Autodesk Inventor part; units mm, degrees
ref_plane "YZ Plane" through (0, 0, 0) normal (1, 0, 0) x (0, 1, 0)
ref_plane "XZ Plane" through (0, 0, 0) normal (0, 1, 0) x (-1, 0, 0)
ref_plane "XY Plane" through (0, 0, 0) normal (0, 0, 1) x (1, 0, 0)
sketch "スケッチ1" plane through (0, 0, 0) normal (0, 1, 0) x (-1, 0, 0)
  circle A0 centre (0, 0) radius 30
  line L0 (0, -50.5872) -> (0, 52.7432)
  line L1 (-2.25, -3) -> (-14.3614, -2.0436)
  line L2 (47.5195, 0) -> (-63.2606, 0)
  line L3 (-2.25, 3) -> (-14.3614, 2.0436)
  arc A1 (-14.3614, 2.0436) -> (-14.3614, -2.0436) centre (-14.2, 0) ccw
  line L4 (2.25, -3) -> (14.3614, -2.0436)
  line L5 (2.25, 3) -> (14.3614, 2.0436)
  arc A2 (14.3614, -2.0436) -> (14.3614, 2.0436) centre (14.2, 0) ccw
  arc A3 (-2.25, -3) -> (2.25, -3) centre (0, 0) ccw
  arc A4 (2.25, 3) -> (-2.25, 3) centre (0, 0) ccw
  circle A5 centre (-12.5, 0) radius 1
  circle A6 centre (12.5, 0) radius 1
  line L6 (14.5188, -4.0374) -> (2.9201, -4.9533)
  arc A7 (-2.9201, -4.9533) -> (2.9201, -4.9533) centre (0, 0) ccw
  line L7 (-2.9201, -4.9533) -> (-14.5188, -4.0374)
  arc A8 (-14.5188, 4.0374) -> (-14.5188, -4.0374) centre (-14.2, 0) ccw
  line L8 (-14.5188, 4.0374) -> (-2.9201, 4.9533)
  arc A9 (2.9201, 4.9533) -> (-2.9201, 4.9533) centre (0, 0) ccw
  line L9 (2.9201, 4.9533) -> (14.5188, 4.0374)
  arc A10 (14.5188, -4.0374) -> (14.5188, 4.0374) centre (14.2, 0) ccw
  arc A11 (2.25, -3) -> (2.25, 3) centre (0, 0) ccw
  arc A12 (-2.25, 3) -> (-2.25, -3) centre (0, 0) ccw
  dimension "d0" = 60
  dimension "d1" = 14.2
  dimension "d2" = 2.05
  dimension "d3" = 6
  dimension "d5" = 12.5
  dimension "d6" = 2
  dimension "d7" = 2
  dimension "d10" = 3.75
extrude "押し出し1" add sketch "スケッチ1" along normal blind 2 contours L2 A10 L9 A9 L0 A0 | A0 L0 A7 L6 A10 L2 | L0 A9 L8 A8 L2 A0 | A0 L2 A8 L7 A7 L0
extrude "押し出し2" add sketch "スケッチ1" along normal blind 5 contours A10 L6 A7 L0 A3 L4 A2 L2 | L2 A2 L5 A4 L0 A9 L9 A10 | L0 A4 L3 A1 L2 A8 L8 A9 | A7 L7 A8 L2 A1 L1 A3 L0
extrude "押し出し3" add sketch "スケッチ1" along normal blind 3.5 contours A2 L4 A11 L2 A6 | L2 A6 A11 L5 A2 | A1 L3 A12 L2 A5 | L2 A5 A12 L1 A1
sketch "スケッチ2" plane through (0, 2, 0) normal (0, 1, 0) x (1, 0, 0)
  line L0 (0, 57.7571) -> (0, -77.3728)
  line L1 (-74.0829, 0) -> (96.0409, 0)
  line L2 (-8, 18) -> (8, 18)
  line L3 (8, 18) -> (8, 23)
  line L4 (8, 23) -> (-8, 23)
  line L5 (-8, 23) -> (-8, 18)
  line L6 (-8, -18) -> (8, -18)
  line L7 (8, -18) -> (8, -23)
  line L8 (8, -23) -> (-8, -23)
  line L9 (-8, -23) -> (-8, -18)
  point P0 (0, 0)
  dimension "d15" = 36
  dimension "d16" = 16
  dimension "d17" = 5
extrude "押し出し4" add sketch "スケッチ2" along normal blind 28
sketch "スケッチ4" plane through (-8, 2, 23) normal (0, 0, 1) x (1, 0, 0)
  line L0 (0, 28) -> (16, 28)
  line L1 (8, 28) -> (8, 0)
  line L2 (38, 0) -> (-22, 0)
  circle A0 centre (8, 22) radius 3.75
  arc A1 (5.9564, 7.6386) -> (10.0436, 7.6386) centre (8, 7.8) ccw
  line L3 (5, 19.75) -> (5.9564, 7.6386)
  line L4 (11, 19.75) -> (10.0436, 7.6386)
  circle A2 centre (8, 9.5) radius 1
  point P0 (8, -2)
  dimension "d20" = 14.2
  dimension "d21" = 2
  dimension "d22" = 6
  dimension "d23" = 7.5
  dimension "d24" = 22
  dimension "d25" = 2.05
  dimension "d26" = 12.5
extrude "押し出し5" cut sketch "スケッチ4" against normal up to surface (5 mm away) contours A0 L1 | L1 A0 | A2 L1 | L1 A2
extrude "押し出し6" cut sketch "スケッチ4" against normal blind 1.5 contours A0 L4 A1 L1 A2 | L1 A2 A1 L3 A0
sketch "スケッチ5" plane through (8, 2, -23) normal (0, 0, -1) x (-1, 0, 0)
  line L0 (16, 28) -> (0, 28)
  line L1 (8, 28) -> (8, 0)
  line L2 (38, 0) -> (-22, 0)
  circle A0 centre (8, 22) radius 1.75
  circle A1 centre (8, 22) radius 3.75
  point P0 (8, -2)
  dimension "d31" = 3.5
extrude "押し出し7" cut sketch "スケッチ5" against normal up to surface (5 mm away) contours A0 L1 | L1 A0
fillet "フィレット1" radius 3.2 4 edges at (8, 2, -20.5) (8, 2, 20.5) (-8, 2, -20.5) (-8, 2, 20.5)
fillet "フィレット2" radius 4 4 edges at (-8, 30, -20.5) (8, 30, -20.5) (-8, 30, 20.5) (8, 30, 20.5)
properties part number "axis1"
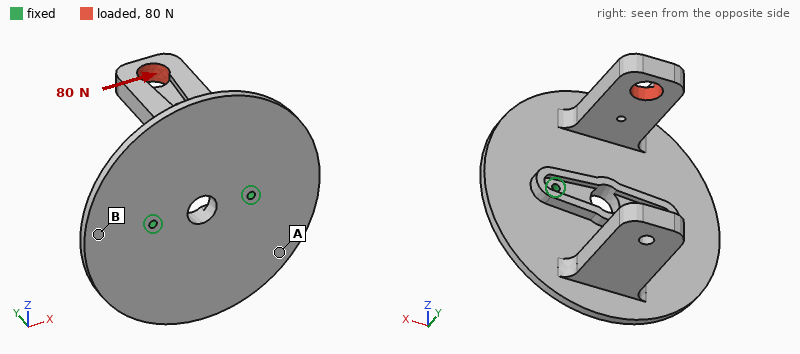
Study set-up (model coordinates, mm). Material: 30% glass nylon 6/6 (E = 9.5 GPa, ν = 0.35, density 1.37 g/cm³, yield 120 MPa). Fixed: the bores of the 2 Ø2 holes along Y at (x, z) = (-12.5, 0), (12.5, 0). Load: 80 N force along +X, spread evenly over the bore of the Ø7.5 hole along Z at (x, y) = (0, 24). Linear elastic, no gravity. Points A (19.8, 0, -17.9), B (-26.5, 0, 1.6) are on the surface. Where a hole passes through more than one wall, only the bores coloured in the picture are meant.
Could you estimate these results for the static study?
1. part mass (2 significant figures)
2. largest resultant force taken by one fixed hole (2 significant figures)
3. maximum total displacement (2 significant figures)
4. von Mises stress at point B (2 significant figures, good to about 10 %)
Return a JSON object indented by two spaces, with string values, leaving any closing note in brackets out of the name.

{
  "part mass": "14 g",
  "largest resultant force taken by one fixed hole": "100 N",
  "maximum total displacement": "0.87 mm",
  "von Mises stress at point B": "13 MPa"
}
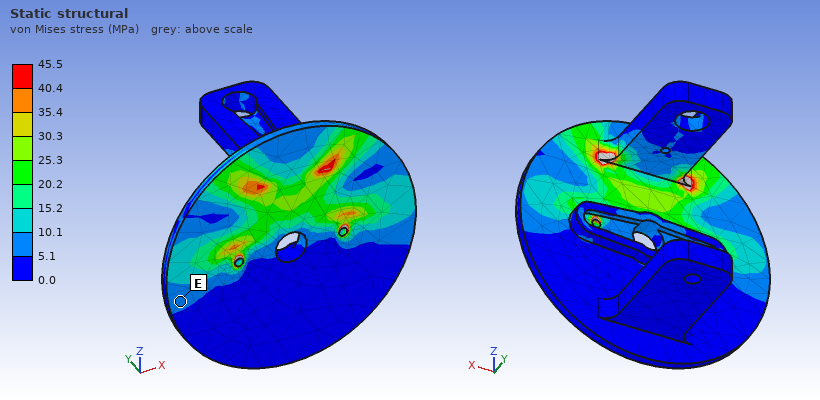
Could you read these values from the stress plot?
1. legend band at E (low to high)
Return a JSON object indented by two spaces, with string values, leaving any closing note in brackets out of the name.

{
  "legend band at E": "5.1 to 10.1 MPa"
}
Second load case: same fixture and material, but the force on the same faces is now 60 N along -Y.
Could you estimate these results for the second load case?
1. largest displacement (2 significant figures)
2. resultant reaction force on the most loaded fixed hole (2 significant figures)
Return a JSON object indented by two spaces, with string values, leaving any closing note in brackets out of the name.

{
  "largest displacement": "1.0 mm",
  "resultant reaction force on the most loaded fixed hole": "30 N"
}
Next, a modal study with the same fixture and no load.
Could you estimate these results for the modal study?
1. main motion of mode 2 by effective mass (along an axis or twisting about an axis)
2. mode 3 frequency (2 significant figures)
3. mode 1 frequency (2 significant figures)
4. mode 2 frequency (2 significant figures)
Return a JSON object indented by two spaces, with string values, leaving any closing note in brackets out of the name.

{
  "main motion of mode 2 by effective mass": "along Y",
  "mode 3 frequency": "1200 Hz",
  "mode 1 frequency": "570 Hz",
  "mode 2 frequency": "640 Hz"
}
